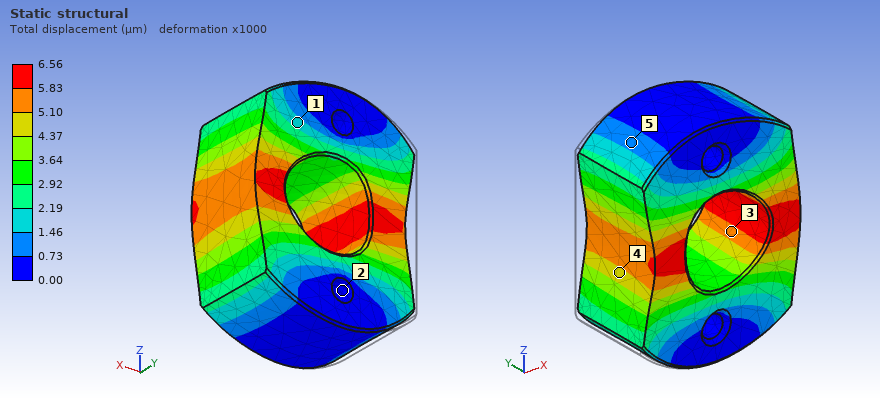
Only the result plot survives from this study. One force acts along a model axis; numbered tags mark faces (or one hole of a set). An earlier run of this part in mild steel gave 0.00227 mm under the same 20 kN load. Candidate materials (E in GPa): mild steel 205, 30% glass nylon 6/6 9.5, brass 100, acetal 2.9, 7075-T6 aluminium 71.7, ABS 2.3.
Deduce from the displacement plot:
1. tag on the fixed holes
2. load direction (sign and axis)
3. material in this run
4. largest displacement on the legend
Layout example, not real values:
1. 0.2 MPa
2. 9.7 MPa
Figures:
1. 2
2. +X
3. 7075-T6 aluminium
4. 6.56 µm
